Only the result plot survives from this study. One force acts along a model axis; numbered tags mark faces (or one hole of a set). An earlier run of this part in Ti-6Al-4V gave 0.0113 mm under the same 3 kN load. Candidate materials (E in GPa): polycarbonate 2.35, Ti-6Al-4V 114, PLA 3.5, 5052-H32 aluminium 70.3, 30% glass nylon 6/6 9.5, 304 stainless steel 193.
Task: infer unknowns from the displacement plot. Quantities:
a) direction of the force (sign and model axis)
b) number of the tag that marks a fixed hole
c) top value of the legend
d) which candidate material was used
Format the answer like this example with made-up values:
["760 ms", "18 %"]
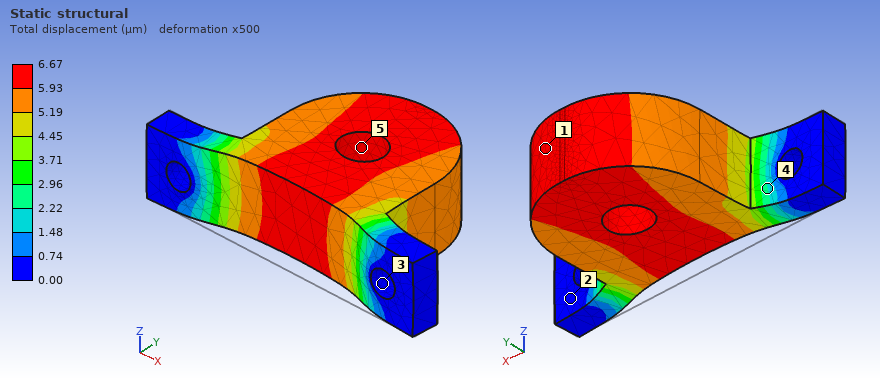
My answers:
["+Y", "3", "6.67 µm", "304 stainless steel"]
